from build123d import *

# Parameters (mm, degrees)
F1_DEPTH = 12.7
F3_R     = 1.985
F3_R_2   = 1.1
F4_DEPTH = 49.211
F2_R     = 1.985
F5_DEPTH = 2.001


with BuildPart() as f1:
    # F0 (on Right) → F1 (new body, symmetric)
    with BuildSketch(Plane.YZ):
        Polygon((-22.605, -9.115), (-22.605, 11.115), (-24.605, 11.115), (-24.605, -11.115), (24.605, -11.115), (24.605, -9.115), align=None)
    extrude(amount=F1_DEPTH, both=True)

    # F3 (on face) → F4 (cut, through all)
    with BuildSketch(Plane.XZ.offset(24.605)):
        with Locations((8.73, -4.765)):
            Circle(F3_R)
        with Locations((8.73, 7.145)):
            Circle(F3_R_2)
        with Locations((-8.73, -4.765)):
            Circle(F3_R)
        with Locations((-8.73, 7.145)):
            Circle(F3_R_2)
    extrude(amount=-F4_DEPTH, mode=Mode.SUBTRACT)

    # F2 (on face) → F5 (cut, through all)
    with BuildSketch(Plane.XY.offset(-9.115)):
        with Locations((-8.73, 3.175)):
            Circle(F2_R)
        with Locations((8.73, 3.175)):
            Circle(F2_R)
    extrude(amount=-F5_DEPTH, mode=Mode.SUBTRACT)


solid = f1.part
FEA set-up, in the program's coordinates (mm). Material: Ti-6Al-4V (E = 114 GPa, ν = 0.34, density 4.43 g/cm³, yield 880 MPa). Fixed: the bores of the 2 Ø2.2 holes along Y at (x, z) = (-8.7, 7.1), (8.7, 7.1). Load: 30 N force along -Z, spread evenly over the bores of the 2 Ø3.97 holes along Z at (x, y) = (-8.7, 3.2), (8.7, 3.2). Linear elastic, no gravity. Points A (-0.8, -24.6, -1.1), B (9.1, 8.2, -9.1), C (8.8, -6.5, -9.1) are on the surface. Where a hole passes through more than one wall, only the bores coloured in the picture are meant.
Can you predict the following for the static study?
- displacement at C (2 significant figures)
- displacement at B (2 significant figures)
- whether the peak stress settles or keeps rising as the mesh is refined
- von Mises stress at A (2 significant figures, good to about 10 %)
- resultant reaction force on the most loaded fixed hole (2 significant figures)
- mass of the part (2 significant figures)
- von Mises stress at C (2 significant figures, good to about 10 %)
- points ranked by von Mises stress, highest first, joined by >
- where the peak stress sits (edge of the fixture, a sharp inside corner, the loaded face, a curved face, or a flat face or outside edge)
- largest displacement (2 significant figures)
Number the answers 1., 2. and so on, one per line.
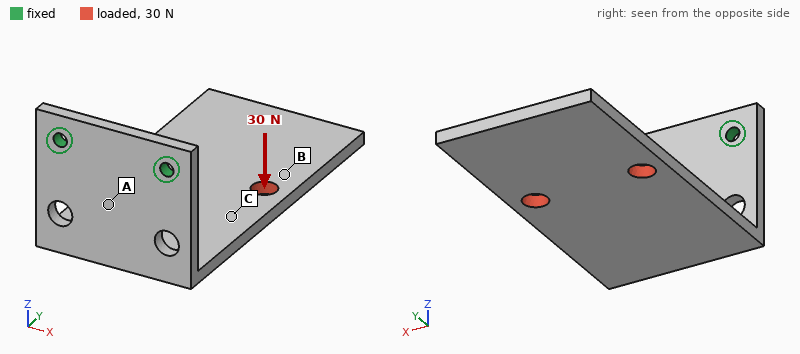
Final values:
1. 0.18 mm
2. 0.37 mm
3. keeps rising
4. 46 MPa
5. 17 N
6. 15 g
7. 17 MPa
8. A > C > B
9. edge of the fixture
10. 0.58 mm
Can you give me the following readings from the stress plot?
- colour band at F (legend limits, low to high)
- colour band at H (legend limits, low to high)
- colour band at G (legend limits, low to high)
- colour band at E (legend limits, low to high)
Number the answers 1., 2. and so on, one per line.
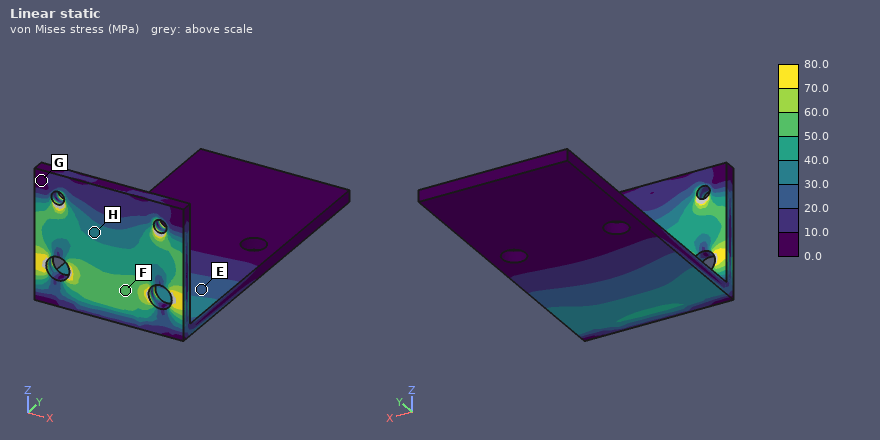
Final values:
1. 50.0 to 60.0 MPa
2. 30.0 to 40.0 MPa
3. 0.0 to 10.0 MPa
4. 20.0 to 30.0 MPa
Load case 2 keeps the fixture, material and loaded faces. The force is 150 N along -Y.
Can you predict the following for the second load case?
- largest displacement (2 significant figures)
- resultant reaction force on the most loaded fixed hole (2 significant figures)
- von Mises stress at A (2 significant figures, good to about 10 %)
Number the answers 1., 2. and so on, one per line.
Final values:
1. 0.63 mm
2. 75 N
3. 76 MPa
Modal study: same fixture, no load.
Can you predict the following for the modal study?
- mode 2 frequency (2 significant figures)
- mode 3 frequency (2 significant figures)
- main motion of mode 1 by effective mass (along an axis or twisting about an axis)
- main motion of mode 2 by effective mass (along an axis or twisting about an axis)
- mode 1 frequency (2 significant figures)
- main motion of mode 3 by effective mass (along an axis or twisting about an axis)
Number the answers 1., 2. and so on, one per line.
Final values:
1. 920 Hz
2. 2000 Hz
3. along Z
4. along X
5. 440 Hz
6. along Y
